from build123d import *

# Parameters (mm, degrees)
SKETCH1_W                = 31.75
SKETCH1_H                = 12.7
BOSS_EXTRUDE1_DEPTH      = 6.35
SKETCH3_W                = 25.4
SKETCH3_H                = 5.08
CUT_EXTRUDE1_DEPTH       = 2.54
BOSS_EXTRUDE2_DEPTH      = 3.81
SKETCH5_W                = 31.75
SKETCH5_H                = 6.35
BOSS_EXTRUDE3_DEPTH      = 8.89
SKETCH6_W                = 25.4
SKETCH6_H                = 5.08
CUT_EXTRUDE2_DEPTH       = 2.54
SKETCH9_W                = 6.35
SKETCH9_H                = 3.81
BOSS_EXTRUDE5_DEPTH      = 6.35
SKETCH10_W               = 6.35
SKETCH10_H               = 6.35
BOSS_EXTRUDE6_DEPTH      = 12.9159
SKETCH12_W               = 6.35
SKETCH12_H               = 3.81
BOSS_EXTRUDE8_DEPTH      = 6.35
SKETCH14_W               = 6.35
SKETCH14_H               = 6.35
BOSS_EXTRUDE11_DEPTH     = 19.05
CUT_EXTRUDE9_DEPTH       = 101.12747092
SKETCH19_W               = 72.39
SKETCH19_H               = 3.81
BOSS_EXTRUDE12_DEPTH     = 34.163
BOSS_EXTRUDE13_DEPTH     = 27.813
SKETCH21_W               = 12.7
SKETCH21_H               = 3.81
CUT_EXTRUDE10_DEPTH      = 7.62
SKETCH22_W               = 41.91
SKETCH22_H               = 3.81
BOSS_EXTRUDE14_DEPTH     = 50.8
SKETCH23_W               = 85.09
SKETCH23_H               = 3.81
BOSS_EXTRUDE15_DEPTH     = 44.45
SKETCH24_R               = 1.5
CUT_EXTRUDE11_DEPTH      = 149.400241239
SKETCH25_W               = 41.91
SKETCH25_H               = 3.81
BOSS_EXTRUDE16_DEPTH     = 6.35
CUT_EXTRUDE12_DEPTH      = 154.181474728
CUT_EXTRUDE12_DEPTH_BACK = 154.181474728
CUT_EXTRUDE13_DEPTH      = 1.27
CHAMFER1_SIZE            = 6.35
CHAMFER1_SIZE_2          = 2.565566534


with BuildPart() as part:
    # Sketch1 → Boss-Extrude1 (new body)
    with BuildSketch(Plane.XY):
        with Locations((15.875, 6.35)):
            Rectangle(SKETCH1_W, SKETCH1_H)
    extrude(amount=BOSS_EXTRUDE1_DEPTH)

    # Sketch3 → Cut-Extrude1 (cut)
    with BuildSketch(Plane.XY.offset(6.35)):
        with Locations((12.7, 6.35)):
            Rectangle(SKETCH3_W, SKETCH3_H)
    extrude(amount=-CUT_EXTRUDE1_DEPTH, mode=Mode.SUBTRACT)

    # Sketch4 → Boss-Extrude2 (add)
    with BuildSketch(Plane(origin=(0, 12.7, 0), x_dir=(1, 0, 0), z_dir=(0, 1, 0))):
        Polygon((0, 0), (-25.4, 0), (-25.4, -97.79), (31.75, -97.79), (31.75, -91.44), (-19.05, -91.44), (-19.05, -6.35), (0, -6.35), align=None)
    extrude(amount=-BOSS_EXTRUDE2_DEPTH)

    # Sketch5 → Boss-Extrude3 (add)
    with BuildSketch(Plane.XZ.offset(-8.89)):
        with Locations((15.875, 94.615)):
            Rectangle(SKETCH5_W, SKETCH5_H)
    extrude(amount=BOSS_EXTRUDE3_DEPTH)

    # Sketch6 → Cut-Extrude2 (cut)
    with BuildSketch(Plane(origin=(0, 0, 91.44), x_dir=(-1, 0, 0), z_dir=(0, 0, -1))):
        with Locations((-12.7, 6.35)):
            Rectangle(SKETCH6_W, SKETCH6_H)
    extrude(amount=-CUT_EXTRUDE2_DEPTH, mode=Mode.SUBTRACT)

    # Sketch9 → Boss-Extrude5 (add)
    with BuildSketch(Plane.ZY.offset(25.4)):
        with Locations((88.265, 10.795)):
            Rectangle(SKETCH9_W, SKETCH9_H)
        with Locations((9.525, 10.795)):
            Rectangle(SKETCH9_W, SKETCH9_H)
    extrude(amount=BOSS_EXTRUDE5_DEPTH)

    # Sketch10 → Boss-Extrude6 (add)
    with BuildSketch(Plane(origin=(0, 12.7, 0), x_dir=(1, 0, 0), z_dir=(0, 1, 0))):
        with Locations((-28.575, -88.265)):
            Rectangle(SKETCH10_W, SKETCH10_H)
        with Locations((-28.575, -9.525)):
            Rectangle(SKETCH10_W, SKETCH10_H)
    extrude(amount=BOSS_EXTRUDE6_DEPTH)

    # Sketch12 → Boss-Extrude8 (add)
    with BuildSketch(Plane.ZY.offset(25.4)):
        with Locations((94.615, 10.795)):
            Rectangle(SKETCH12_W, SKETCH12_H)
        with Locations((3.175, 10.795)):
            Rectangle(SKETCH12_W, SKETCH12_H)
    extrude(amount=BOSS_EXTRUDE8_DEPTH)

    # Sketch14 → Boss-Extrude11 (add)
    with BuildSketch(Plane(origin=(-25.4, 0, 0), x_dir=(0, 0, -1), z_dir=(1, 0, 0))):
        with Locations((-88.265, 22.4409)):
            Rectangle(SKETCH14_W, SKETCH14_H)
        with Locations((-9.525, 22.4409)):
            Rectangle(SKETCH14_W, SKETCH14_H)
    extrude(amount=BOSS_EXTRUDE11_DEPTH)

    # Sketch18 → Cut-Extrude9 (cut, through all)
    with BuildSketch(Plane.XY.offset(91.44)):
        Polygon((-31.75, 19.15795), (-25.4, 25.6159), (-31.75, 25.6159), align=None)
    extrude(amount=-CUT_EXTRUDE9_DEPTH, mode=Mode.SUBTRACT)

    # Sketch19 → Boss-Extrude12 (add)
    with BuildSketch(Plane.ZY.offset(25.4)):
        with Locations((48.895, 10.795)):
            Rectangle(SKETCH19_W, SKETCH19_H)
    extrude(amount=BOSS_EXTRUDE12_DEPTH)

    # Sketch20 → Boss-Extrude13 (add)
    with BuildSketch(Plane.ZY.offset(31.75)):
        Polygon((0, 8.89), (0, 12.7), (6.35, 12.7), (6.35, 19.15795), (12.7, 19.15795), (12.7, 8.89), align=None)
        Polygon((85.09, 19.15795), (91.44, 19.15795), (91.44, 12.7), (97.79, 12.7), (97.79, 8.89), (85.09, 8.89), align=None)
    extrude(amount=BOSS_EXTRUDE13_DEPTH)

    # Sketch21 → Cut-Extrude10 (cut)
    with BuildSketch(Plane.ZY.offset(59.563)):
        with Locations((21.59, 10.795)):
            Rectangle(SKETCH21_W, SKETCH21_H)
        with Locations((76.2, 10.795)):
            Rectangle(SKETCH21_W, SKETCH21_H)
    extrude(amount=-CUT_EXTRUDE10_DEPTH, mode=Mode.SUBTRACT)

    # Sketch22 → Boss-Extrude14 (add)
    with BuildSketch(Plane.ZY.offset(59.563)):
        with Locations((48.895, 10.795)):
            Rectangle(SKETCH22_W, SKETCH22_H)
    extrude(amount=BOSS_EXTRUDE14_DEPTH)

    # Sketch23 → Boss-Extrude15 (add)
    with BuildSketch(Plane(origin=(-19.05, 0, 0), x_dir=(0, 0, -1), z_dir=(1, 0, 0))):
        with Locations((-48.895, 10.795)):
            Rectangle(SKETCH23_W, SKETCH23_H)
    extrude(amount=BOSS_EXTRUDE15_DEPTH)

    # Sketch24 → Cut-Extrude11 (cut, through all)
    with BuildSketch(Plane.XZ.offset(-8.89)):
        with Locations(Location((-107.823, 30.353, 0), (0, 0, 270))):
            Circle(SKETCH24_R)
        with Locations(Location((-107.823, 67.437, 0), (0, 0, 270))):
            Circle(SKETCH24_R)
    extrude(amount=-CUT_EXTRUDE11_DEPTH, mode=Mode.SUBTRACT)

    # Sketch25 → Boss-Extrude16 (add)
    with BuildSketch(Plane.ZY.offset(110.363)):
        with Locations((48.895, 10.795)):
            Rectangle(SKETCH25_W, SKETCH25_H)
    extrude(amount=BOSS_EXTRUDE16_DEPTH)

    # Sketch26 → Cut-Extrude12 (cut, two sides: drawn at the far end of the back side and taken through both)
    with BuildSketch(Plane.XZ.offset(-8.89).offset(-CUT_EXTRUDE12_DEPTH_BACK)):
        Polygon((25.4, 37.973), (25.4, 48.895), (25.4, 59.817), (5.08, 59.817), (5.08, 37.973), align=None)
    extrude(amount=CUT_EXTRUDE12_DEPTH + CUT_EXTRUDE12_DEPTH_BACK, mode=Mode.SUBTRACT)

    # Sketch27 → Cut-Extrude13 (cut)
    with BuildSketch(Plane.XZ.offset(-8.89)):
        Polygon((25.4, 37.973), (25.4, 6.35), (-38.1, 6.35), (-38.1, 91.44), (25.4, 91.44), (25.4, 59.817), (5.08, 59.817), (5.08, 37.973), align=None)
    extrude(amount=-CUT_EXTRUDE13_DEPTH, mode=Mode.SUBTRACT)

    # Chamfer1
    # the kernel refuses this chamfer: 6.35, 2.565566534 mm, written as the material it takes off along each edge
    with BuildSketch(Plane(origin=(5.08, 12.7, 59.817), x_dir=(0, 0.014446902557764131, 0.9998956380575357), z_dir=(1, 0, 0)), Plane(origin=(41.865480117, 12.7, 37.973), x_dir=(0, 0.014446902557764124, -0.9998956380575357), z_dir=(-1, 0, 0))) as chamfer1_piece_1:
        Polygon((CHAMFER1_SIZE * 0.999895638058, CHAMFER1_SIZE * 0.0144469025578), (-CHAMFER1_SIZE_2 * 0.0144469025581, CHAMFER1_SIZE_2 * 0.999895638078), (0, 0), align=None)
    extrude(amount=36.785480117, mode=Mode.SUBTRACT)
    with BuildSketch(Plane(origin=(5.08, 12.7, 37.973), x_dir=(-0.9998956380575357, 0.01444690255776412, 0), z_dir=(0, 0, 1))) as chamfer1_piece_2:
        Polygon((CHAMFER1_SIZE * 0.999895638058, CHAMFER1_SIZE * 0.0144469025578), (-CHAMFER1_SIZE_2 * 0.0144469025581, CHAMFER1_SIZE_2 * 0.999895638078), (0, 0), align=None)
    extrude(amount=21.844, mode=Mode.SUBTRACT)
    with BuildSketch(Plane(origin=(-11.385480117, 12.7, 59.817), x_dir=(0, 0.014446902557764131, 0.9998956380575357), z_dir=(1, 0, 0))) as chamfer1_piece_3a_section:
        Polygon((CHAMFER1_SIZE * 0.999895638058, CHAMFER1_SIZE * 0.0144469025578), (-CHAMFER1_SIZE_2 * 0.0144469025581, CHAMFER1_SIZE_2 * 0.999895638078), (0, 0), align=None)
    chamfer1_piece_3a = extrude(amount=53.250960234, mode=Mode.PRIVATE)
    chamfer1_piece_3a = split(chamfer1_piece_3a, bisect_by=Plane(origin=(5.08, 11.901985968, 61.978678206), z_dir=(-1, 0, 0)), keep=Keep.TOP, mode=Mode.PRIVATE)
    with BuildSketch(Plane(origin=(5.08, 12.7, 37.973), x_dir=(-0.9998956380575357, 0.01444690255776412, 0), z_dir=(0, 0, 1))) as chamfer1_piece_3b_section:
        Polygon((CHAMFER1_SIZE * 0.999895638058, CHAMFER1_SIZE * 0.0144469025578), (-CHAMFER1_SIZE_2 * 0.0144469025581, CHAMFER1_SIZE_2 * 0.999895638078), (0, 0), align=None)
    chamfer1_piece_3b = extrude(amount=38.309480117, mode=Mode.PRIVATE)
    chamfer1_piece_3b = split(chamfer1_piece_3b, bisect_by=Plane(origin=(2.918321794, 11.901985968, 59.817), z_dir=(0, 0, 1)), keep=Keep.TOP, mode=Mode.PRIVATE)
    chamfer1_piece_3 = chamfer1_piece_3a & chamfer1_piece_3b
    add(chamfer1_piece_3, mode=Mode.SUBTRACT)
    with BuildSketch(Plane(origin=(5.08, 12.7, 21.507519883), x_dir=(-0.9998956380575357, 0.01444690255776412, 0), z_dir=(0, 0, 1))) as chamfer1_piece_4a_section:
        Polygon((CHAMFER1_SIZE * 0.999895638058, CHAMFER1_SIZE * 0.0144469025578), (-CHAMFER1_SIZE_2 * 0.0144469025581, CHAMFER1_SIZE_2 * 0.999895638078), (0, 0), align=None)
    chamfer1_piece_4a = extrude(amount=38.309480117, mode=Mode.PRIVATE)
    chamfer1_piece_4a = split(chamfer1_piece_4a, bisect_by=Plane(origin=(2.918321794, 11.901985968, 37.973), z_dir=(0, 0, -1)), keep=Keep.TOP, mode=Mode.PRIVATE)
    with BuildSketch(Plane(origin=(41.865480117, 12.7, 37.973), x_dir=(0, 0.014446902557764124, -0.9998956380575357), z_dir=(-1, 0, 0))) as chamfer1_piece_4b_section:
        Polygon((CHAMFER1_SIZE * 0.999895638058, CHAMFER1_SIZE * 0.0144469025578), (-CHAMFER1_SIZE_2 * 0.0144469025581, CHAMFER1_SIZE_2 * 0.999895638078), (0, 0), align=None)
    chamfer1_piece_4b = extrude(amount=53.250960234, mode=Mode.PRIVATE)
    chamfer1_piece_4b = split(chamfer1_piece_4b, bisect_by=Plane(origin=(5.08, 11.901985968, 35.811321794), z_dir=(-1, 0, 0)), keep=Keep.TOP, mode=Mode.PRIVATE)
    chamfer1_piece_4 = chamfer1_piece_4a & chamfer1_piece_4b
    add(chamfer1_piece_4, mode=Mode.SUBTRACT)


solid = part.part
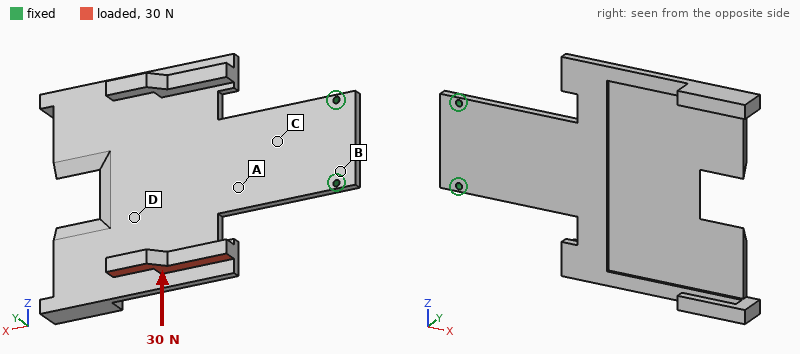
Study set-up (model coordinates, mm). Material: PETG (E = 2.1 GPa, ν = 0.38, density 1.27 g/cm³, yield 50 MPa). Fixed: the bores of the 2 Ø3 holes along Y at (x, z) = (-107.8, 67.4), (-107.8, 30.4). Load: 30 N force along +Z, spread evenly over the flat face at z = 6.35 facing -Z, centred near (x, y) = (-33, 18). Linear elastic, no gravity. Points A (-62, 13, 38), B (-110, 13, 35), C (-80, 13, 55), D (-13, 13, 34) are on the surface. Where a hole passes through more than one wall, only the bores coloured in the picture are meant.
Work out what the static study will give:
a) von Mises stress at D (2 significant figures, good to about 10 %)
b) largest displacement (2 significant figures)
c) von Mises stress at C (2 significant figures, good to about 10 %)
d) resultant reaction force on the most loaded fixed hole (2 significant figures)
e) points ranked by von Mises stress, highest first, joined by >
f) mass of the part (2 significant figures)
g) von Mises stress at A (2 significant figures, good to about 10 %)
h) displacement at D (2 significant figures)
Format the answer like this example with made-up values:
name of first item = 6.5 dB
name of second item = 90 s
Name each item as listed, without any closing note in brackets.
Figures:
von Mises stress at D = 1.6 MPa
largest displacement = 1.7 mm
von Mises stress at C = 2.2 MPa
resultant reaction force on the most loaded fixed hole = 63 N
points ranked by von Mises stress, highest first, joined by > = A > C > D > B
mass of the part = 50 g
von Mises stress at A = 2.8 MPa
displacement at D = 0.36 mm
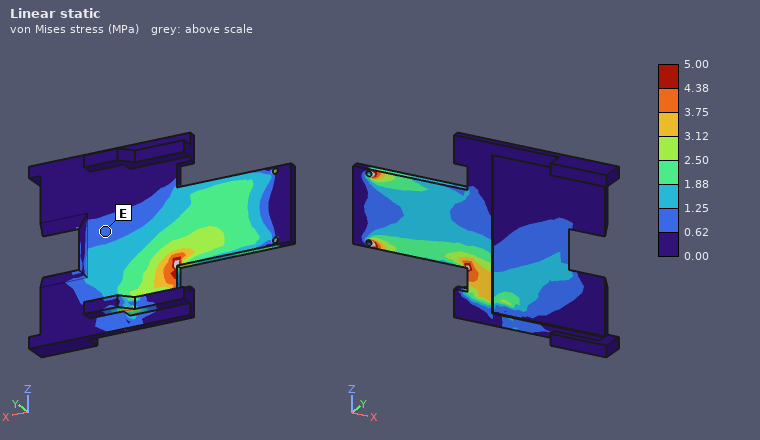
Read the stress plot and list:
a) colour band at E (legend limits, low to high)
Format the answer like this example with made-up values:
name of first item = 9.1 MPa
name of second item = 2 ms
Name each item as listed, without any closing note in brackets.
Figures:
colour band at E = 0.62 to 1.25 MPa
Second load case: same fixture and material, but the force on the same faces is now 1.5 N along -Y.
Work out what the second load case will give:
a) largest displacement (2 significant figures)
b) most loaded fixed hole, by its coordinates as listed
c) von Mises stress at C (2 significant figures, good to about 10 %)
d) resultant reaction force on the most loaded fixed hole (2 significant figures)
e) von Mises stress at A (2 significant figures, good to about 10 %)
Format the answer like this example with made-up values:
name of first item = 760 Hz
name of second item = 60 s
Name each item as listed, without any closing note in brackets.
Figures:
largest displacement = 1.8 mm
most loaded fixed hole, by its coordinates as listed = (-107.8, 30.4)
von Mises stress at C = 0.81 MPa
resultant reaction force on the most loaded fixed hole = 2.6 N
von Mises stress at A = 0.76 MPa
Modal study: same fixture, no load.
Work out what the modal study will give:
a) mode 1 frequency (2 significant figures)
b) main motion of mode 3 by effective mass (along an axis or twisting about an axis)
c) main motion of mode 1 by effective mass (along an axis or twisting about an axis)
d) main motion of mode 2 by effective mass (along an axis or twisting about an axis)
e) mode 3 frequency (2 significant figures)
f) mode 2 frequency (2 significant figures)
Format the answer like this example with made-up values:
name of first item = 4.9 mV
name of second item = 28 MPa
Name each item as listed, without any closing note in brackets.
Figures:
mode 1 frequency = 29 Hz
main motion of mode 3 by effective mass = along Y
main motion of mode 1 by effective mass = along Y
main motion of mode 2 by effective mass = twisting about X
mode 3 frequency = 170 Hz
mode 2 frequency = 64 Hz
